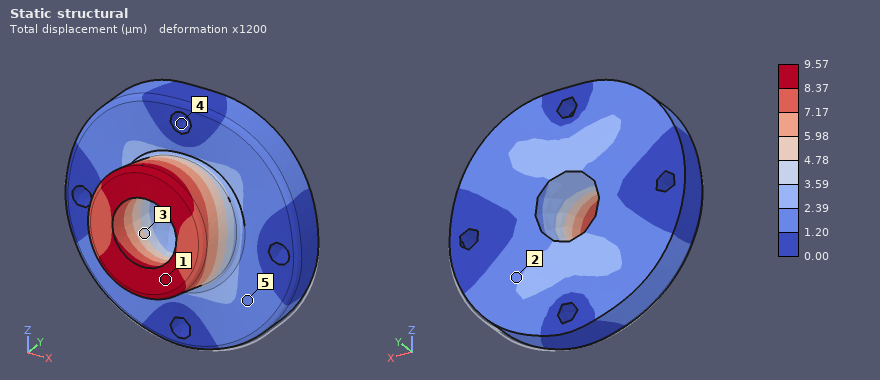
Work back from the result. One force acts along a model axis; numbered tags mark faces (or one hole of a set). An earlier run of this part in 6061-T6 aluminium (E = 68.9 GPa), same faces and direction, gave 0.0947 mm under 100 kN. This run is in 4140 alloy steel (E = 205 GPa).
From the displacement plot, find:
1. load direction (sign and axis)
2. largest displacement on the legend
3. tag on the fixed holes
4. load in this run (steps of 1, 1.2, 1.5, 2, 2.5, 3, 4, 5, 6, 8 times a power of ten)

+Z
9.57 µm
4
30 kN
